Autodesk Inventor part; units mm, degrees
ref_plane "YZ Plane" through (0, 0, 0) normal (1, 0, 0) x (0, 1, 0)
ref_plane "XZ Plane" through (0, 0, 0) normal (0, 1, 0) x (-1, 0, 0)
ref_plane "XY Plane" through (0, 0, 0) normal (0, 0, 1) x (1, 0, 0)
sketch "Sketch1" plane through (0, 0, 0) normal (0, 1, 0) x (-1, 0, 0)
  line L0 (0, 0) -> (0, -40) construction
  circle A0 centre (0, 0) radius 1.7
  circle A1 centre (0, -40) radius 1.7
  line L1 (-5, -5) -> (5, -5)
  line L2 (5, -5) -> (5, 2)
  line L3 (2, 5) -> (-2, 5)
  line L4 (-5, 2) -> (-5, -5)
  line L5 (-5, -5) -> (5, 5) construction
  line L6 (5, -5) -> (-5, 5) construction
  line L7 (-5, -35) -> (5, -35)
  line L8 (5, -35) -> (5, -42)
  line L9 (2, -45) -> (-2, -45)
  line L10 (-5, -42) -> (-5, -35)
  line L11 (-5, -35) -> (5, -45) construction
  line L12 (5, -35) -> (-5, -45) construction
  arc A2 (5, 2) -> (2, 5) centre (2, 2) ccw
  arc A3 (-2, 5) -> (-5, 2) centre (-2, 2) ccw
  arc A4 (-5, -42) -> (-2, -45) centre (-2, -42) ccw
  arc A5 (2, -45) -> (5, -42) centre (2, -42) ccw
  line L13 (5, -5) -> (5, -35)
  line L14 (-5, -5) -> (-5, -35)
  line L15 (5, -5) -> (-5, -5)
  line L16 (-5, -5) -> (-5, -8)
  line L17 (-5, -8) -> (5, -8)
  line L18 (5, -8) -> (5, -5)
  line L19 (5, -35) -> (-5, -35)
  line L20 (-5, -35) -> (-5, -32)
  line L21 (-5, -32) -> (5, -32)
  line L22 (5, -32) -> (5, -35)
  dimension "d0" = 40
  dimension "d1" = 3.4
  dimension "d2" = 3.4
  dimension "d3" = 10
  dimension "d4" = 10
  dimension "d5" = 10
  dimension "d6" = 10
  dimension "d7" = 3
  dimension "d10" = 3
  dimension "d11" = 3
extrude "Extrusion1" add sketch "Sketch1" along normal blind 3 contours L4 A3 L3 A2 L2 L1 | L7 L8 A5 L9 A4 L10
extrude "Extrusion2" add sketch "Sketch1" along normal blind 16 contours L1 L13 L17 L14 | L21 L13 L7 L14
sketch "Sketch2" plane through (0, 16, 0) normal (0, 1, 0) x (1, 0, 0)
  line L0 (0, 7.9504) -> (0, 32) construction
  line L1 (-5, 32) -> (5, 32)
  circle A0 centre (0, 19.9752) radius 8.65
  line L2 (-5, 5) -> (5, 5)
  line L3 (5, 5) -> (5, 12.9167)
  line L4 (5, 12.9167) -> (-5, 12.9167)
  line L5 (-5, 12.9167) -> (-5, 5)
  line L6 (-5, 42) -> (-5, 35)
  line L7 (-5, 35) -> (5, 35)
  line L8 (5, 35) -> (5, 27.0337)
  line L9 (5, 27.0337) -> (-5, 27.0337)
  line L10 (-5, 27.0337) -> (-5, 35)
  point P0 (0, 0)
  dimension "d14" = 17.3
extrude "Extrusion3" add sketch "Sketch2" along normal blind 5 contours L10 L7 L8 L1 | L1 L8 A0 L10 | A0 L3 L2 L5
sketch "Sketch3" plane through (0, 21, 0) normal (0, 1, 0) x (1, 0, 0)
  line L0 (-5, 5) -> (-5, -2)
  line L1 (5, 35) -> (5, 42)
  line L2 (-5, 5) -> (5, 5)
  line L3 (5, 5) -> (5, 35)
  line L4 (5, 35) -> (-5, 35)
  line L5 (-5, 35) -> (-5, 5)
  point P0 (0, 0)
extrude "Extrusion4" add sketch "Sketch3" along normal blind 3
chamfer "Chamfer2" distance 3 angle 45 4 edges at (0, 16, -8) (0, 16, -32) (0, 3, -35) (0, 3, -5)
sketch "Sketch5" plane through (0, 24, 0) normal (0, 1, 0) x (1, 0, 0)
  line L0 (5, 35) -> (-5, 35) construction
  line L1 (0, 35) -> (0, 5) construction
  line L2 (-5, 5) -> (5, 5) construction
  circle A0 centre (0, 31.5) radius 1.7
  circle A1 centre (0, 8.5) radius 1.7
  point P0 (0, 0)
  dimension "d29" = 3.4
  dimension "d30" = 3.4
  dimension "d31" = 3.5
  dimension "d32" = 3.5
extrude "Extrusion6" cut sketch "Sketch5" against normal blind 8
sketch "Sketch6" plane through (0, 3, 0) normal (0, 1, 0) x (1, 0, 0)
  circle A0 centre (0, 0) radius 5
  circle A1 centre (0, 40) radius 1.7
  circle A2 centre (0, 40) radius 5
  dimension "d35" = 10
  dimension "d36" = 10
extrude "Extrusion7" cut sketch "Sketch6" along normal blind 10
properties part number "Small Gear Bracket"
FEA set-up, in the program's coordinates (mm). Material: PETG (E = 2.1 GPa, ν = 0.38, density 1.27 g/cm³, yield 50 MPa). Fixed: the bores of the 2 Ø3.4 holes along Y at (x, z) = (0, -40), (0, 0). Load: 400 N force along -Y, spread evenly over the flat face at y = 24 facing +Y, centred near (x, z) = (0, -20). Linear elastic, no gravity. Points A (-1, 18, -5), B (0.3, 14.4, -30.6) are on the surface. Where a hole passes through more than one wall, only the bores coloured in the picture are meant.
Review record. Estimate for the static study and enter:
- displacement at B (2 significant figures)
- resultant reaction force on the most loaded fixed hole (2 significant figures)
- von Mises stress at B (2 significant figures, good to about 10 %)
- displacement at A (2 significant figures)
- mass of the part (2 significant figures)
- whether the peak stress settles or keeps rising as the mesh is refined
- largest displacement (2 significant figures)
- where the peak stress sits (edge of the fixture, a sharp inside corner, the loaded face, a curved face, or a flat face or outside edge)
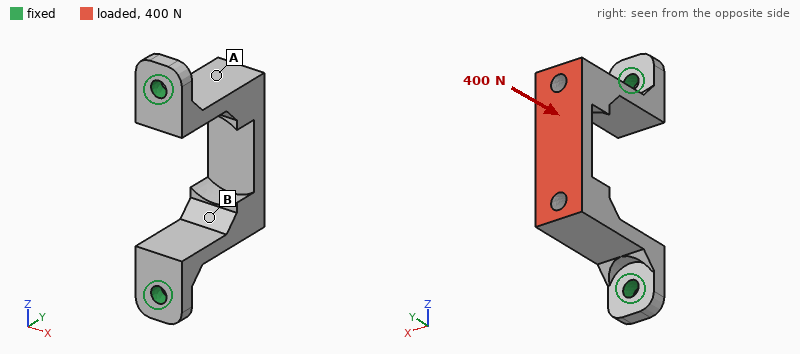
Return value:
0.17 mm
210 N
14 MPa
0.14 mm
3.9 g
keeps rising
0.37 mm
edge of the fixture
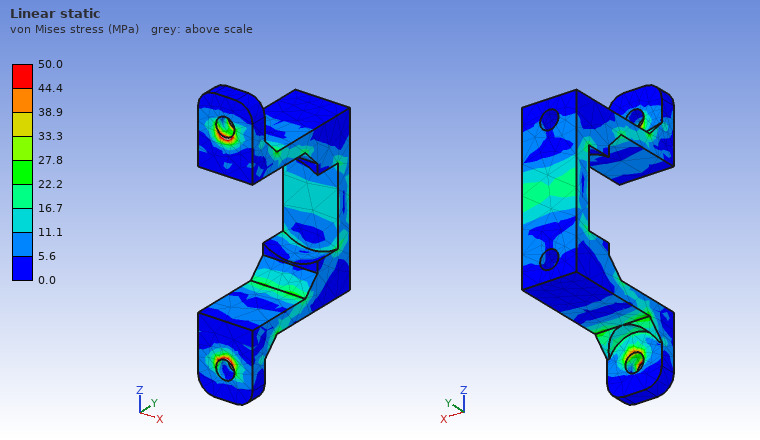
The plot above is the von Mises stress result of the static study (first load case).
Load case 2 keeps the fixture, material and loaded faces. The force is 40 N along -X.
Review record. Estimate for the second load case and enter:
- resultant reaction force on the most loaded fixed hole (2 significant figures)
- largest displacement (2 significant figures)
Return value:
20 N
0.66 mm
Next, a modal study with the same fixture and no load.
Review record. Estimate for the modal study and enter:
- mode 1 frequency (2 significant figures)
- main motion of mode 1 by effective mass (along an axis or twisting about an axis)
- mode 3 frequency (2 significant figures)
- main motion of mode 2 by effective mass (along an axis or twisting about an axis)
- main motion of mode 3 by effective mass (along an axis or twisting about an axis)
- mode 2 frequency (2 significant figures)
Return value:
1000 Hz
along X
1800 Hz
along Z
twisting about Y
1500 Hz
